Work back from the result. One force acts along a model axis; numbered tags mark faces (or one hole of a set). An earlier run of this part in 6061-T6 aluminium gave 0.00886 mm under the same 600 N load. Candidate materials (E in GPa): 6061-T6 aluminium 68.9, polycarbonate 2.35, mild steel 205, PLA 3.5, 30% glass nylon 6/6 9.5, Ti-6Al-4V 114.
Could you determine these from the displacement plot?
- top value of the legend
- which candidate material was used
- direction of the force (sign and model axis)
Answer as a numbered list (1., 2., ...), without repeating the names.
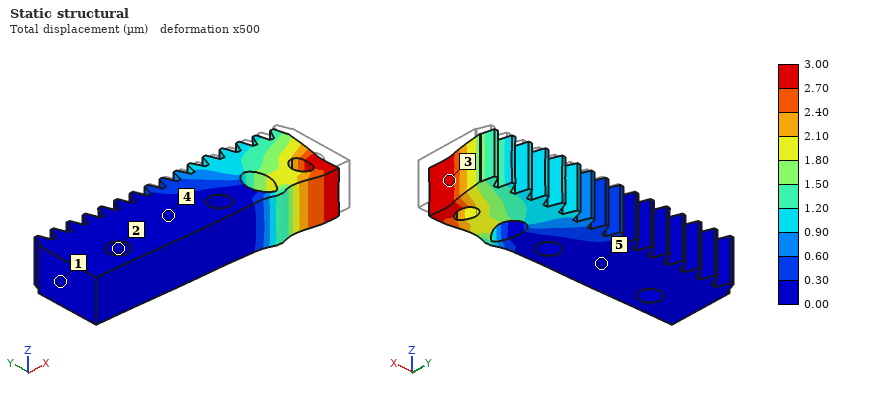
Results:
1. 3.00 µm
2. mild steel
3. -X
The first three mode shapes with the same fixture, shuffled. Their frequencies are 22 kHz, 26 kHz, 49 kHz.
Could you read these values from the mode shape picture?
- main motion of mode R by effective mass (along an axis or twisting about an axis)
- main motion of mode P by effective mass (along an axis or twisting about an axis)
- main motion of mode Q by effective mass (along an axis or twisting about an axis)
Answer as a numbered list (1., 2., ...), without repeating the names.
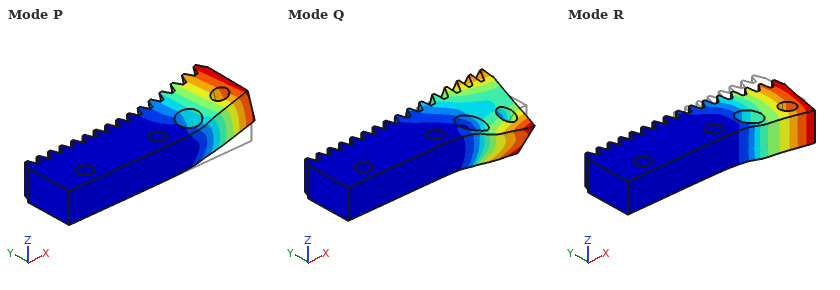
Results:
1. along Y
2. along Z
3. twisting about X
